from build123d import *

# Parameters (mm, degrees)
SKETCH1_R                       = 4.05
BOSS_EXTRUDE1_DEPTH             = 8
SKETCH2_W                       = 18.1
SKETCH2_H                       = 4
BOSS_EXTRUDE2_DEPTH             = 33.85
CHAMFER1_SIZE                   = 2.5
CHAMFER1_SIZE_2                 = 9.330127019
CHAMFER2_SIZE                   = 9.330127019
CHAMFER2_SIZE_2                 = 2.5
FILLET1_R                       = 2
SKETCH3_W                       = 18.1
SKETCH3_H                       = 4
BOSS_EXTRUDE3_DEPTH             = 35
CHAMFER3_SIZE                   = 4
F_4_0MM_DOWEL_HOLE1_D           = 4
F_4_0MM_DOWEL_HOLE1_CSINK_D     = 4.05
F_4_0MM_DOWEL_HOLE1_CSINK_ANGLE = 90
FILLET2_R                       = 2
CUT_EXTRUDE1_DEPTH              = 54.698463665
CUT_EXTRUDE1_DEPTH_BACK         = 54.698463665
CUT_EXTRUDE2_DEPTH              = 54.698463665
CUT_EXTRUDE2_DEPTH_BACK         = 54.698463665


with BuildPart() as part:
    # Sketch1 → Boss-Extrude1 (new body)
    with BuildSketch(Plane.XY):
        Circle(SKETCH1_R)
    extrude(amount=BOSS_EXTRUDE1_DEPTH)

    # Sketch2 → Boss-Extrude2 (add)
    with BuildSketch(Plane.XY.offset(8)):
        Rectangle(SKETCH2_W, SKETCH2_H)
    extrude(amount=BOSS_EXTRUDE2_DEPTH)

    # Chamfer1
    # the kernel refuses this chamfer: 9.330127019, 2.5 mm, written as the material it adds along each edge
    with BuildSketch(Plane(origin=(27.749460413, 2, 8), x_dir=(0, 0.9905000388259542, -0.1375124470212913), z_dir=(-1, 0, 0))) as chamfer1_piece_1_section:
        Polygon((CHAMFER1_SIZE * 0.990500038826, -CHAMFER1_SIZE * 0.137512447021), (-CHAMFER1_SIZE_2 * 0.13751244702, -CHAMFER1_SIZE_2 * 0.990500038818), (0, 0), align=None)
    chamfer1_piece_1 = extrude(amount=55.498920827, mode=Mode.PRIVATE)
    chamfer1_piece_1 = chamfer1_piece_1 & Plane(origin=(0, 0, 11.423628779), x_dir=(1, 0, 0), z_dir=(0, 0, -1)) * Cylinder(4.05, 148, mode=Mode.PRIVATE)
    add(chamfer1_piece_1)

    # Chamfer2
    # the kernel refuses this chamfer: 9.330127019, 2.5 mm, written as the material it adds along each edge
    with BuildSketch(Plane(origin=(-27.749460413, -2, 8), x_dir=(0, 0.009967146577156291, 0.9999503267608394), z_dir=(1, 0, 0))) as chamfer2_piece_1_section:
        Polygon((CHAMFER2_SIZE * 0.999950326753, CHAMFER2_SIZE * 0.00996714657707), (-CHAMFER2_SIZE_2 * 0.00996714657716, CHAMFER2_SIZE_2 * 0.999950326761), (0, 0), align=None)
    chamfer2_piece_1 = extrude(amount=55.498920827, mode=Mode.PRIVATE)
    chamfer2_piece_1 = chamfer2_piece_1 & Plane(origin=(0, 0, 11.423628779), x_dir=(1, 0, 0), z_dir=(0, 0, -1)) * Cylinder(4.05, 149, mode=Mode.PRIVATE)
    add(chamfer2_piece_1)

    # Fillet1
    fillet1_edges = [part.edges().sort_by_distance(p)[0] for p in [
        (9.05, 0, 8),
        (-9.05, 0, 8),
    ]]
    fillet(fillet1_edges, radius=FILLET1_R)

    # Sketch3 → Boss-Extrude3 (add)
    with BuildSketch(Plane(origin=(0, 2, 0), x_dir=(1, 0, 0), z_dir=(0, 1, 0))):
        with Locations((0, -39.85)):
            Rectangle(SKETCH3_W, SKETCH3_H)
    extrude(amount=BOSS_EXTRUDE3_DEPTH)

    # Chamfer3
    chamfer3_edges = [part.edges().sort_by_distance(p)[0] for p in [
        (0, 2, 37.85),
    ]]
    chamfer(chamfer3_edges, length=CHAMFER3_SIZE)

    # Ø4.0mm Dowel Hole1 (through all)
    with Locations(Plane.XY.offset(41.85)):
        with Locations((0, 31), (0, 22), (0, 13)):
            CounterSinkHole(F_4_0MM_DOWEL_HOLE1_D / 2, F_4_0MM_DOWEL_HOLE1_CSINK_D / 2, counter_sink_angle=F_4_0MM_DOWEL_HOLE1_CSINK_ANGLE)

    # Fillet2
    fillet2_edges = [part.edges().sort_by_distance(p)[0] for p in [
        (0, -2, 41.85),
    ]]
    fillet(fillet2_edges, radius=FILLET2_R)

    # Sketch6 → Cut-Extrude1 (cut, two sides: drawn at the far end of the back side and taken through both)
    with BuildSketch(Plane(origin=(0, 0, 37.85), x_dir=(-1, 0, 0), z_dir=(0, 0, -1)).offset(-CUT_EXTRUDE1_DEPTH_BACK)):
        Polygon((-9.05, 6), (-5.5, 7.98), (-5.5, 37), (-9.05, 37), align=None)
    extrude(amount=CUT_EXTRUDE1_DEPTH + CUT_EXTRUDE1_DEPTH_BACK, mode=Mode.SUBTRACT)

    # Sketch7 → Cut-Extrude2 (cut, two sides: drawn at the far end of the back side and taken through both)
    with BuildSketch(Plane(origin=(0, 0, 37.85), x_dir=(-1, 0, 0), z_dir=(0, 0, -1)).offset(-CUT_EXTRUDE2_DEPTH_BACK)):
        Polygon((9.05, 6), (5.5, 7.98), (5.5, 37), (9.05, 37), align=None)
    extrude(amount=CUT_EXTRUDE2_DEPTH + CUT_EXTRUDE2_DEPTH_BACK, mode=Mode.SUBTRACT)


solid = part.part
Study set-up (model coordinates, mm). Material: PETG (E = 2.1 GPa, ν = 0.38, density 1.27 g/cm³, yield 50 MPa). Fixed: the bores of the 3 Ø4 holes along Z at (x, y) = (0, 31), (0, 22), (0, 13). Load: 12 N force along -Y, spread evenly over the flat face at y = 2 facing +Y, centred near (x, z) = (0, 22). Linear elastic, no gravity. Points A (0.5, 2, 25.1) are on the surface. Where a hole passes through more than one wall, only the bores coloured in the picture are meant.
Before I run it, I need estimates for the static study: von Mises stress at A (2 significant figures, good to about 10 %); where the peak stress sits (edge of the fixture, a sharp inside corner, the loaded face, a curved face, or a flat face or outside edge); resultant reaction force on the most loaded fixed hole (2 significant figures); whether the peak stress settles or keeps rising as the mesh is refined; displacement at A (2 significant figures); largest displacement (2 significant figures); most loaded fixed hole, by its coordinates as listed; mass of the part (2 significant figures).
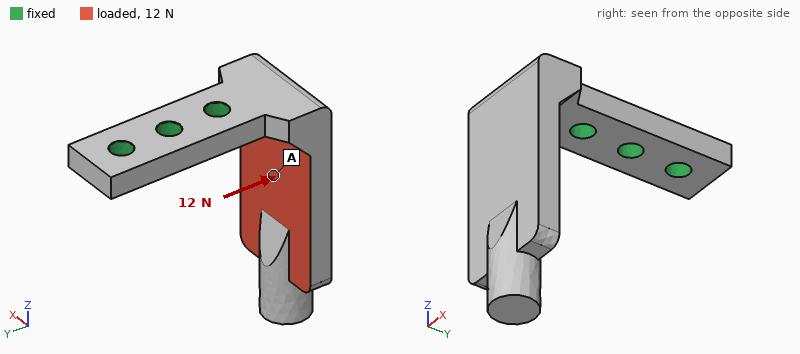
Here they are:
1.1 MPa
edge of the fixture
11 N
keeps rising
0.23 mm
0.71 mm
(0, 13)
5.9 g
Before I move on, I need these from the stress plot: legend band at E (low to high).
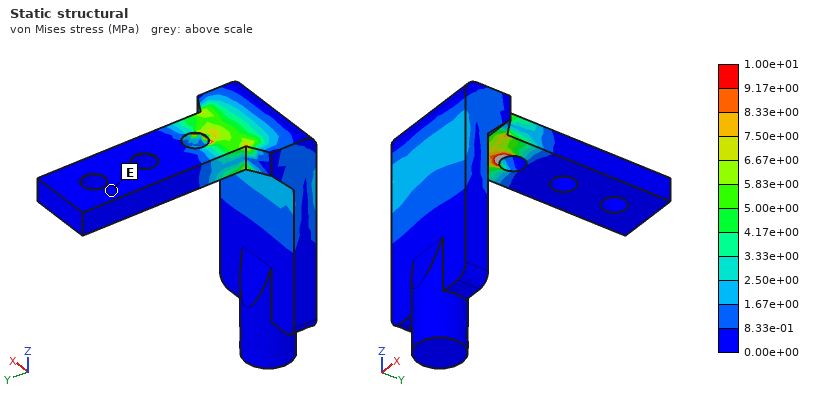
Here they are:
0.00e+00 to 8.33e-01 MPa
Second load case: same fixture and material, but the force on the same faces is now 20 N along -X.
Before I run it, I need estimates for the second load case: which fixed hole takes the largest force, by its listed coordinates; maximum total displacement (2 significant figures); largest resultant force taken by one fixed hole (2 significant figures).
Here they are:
(0, 13)
0.64 mm
28 N
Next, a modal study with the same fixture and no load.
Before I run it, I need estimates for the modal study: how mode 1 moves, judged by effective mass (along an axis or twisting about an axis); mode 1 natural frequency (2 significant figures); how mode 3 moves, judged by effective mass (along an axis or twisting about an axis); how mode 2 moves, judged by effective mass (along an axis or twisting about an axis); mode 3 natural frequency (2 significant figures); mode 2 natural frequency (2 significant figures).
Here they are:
along Y
390 Hz
along Z
along X
1700 Hz
550 Hz
